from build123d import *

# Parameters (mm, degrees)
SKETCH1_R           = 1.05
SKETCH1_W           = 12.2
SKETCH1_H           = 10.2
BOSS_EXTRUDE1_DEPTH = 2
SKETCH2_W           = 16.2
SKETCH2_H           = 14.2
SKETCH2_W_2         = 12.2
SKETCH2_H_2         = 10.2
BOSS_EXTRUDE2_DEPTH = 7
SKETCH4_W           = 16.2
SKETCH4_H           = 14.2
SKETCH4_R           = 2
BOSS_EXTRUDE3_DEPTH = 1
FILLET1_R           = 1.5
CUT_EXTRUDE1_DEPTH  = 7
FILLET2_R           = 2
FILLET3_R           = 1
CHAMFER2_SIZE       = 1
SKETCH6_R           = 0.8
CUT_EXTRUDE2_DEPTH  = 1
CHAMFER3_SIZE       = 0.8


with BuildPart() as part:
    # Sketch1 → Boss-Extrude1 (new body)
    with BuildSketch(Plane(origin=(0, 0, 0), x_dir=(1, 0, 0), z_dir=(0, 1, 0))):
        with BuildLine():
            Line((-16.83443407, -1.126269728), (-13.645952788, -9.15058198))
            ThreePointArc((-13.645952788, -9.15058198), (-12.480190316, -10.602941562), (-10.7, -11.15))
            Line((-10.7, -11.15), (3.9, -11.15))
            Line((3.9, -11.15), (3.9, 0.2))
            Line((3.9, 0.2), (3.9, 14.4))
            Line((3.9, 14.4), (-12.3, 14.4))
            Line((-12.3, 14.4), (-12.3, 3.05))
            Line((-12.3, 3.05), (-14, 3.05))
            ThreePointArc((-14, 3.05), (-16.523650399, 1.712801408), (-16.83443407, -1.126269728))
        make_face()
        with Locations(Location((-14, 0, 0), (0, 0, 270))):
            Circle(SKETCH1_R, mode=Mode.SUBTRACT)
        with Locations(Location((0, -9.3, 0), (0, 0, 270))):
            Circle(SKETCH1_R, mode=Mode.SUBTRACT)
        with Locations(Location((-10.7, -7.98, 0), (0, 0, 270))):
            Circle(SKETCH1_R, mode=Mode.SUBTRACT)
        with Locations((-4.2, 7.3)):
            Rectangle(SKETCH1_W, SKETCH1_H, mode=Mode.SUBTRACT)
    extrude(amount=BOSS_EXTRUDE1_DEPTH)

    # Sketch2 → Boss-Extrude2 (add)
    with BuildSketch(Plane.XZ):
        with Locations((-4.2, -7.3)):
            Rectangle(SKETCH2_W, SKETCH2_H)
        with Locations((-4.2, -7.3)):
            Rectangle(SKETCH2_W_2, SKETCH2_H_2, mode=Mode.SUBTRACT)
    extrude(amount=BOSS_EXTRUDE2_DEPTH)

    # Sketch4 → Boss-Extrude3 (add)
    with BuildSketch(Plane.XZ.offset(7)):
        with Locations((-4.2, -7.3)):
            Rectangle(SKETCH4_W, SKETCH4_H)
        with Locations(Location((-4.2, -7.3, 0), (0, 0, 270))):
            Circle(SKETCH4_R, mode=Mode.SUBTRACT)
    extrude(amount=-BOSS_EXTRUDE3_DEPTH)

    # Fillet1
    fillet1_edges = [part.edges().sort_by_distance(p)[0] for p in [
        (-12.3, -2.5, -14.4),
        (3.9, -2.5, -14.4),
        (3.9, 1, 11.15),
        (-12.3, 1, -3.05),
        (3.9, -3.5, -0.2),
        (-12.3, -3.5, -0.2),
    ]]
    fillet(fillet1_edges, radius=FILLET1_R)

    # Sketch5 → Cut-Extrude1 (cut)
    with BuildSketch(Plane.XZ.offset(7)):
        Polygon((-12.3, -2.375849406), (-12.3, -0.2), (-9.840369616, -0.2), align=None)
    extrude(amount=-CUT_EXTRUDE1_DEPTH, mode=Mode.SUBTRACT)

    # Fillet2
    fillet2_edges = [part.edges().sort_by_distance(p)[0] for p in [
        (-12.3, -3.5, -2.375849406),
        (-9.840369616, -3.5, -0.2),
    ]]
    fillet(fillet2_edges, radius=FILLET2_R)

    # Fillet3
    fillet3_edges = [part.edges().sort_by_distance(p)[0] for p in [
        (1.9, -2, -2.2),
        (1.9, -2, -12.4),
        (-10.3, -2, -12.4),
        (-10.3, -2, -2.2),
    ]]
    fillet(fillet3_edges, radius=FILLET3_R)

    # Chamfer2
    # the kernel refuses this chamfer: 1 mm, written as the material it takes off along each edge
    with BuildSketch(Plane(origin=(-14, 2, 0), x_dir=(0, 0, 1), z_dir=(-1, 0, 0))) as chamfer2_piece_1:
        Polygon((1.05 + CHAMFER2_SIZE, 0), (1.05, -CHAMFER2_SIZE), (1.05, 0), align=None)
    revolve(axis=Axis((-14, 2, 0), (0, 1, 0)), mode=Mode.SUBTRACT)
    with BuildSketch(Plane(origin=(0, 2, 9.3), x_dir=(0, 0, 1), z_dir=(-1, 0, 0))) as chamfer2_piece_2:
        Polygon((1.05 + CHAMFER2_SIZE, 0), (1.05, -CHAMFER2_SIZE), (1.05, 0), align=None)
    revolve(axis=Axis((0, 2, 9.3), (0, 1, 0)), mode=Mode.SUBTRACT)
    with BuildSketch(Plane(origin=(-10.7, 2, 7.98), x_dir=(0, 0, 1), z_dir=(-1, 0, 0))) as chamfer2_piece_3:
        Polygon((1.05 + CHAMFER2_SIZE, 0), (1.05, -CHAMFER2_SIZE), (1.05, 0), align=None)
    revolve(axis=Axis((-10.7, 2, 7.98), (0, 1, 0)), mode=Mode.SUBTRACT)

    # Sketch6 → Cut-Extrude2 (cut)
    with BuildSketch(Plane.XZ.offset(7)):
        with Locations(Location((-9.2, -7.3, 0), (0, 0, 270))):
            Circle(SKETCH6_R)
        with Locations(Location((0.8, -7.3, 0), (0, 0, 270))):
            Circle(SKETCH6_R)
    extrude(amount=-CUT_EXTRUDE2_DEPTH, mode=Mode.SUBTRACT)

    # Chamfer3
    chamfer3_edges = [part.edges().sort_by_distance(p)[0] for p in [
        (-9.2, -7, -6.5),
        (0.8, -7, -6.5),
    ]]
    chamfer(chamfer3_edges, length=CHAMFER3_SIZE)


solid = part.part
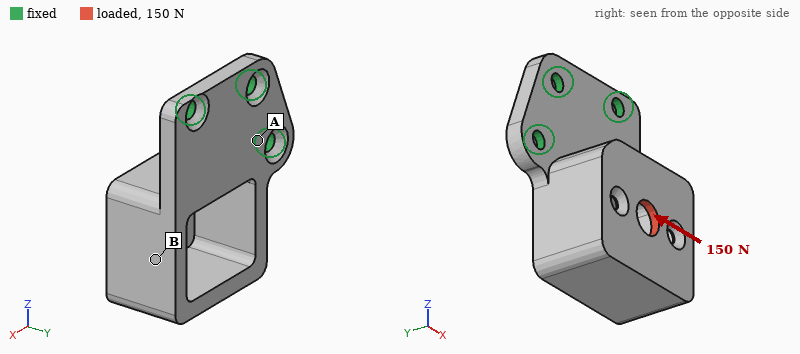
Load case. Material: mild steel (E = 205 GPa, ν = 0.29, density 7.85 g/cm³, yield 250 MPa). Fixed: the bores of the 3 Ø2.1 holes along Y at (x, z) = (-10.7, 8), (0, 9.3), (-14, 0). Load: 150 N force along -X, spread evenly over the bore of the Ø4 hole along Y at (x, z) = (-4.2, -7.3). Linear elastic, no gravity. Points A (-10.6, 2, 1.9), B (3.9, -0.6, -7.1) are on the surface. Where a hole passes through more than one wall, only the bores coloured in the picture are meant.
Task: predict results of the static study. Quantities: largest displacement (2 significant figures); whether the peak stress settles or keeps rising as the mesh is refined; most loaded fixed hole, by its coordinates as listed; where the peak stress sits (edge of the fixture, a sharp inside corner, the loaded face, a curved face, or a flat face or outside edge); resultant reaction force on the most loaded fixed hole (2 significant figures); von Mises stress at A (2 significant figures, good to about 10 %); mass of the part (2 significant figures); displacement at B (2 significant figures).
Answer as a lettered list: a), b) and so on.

a) 30 µm
b) keeps rising
c) (-14, 0)
d) edge of the fixture
e) 180 N
f) 31 MPa
g) 11 g
h) 22 µm
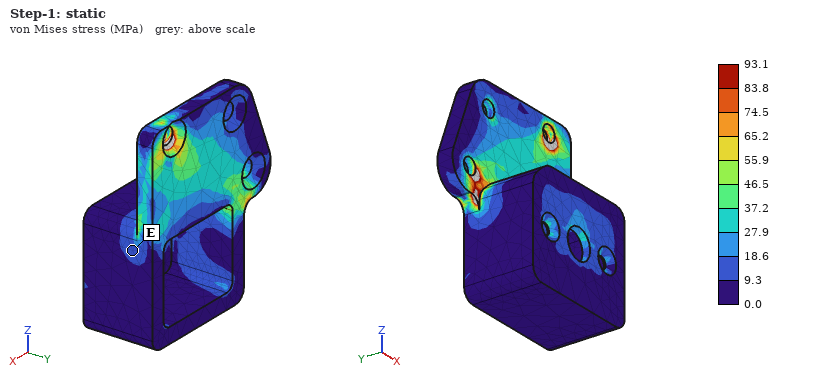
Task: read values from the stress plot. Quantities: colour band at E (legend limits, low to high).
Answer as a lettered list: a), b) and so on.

a) 9.3 to 18.6 MPa
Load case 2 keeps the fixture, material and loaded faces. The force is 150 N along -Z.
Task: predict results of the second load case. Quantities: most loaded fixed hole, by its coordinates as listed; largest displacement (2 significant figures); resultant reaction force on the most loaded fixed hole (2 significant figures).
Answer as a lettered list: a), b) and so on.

a) (0, 9.3)
b) 56 µm
c) 100 N
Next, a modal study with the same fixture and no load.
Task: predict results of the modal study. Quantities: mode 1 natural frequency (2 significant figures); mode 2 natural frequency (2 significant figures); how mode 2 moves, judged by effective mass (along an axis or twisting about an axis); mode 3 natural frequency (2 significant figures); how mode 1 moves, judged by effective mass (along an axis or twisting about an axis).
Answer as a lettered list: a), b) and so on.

a) 2800 Hz
b) 9000 Hz
c) along X
d) 9400 Hz
e) along Y
